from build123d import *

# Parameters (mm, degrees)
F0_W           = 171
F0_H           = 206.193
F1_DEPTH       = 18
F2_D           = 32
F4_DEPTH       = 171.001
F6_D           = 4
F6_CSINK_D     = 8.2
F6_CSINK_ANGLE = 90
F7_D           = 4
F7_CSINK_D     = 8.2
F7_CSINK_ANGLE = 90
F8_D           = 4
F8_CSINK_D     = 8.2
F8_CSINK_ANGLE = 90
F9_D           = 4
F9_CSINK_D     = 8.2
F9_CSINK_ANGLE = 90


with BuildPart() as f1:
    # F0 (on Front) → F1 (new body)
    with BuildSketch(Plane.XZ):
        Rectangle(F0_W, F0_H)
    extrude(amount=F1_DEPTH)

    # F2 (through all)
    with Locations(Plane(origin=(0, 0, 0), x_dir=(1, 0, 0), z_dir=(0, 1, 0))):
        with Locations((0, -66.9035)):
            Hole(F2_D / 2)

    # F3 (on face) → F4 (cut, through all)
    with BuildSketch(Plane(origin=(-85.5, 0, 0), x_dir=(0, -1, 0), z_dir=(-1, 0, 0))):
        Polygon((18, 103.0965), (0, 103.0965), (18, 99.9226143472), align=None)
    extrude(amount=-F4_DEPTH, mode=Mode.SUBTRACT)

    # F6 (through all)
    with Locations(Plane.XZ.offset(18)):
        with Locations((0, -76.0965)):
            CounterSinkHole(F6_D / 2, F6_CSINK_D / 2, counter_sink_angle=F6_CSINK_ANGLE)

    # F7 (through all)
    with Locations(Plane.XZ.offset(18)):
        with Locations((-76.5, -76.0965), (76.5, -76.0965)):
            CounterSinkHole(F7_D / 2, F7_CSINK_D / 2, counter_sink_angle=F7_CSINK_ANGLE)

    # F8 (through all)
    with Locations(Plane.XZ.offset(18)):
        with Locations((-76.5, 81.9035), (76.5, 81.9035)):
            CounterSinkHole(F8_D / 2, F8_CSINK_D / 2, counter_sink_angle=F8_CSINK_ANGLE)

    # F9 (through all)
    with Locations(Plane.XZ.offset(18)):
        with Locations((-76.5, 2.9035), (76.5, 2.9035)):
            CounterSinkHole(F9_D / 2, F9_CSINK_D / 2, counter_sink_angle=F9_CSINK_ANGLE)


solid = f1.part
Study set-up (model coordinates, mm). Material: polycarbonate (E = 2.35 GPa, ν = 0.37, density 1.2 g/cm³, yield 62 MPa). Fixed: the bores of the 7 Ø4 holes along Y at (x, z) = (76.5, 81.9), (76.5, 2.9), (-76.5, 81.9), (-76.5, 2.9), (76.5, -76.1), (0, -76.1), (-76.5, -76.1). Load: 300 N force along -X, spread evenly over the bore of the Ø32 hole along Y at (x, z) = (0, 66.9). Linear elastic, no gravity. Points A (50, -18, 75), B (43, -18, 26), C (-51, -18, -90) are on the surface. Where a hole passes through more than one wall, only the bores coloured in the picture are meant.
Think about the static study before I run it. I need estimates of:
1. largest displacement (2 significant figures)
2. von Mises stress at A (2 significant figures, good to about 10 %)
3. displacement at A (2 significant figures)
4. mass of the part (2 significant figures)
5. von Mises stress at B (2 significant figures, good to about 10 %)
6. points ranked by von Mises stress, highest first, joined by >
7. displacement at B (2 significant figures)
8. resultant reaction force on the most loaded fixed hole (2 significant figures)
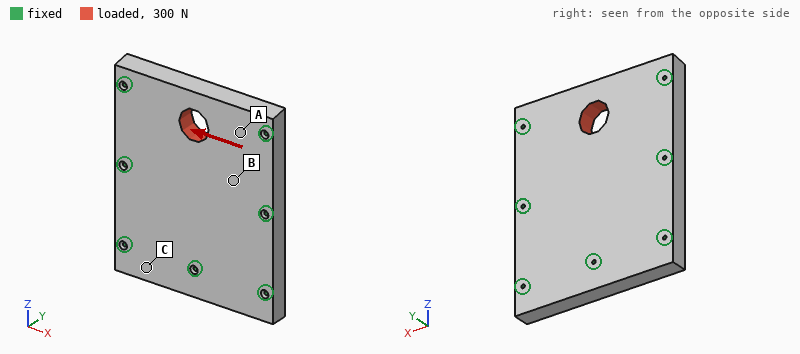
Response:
5.6 µm
0.15 MPa
2.7 µm
740 g
0.076 MPa
A > B > C
2.0 µm
96 N
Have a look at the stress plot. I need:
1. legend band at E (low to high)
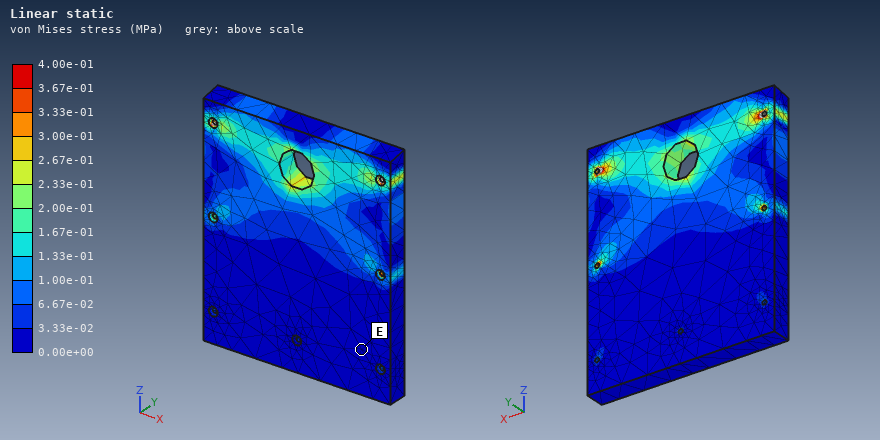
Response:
0.00e+00 to 3.33e-02 MPa
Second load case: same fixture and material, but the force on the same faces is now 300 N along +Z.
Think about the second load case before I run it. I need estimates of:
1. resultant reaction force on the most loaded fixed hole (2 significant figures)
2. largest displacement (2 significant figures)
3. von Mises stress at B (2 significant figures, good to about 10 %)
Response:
66 N
11 µm
0.12 MPa
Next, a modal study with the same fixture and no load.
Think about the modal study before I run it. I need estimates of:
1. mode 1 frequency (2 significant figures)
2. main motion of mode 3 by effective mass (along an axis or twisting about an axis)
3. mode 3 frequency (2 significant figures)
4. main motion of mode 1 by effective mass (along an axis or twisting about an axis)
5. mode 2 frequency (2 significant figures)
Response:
800 Hz
twisting about Z
1900 Hz
along Y
1300 Hz
